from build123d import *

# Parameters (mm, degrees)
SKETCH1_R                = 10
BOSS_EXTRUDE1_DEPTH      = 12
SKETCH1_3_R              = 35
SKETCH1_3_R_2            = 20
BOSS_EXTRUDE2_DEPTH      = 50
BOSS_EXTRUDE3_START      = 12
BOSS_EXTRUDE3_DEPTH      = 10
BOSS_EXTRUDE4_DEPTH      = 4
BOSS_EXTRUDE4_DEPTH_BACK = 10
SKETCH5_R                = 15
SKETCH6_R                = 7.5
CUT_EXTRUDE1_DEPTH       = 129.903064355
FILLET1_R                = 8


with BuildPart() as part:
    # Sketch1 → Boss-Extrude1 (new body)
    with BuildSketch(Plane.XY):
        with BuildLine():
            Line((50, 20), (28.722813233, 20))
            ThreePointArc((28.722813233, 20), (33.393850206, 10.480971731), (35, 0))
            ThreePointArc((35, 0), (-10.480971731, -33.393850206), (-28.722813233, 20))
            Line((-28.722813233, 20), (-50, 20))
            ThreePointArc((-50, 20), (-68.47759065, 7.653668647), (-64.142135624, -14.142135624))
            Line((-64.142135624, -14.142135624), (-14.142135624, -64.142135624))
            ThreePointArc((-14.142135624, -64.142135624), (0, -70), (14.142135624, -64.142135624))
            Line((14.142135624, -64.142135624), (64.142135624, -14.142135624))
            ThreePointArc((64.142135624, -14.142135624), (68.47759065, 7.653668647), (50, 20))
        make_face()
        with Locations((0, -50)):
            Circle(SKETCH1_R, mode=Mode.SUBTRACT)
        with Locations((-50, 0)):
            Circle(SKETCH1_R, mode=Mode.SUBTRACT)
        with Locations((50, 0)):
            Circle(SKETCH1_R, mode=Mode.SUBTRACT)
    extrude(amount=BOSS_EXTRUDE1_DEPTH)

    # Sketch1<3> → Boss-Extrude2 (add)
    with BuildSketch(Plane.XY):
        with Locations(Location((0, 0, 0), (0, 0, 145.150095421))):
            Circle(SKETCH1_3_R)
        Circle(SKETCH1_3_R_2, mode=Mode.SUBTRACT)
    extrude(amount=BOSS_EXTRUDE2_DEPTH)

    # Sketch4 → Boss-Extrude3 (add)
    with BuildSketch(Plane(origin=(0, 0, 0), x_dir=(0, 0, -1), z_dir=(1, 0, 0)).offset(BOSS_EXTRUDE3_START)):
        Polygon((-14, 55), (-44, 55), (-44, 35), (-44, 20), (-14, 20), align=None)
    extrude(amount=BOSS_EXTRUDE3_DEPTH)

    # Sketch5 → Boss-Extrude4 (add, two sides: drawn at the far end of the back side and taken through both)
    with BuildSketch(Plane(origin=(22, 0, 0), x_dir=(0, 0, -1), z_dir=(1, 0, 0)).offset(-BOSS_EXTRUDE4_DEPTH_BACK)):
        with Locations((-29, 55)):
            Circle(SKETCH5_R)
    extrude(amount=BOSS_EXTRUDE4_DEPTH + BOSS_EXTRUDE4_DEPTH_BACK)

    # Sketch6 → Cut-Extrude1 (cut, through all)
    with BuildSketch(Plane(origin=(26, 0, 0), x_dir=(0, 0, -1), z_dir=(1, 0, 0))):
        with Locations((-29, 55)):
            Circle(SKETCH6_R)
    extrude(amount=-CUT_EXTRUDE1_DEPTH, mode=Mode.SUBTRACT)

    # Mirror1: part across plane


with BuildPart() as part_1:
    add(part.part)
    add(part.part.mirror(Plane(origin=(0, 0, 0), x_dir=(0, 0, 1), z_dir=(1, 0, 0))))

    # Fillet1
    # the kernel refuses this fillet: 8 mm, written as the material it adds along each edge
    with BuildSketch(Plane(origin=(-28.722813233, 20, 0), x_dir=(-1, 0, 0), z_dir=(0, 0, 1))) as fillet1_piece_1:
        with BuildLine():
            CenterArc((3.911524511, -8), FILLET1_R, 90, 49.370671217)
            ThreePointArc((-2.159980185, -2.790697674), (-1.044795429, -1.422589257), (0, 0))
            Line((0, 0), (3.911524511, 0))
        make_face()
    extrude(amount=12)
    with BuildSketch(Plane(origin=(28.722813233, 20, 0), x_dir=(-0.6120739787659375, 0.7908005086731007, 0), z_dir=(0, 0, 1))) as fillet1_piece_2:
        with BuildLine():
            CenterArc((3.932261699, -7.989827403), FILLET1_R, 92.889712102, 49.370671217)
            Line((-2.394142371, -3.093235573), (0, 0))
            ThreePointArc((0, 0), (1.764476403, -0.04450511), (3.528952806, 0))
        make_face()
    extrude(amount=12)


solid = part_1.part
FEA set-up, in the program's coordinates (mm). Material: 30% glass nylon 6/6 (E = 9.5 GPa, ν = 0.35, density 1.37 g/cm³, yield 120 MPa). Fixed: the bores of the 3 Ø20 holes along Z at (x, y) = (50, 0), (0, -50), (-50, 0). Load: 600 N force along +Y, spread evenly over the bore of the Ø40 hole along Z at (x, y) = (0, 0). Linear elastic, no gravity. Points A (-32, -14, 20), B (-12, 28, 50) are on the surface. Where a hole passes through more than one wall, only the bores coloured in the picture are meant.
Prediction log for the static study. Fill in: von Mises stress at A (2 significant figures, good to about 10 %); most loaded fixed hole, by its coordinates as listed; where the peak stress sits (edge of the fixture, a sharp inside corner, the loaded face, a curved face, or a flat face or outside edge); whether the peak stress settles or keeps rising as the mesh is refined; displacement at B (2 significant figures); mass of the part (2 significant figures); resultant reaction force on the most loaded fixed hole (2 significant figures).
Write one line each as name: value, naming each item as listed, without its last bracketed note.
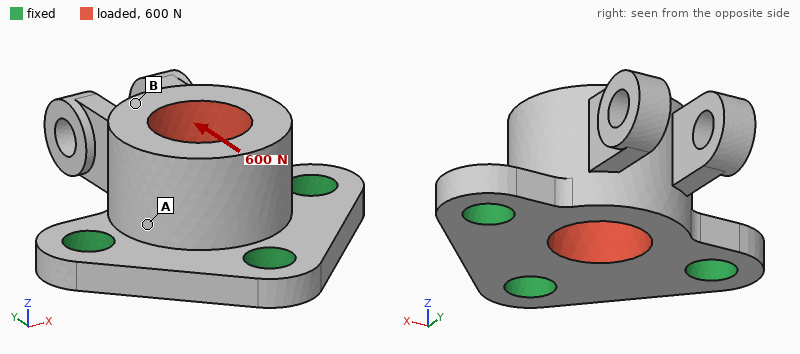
von Mises stress at A: 0.63 MPa
most loaded fixed hole, by its coordinates as listed: (0, -50)
where the peak stress sits: edge of the fixture
whether the peak stress settles or keeps rising as the mesh is refined: keeps rising
displacement at B: 15 µm
mass of the part: 280 g
resultant reaction force on the most loaded fixed hole: 360 N
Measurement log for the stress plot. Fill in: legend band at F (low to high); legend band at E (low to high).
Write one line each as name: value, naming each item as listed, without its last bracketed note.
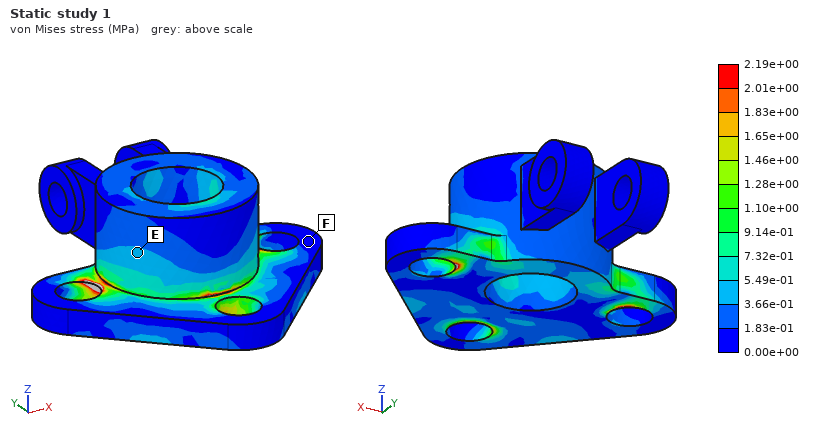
legend band at F: 0.00e+00 to 1.83e-01 MPa
legend band at E: 3.66e-01 to 5.49e-01 MPa
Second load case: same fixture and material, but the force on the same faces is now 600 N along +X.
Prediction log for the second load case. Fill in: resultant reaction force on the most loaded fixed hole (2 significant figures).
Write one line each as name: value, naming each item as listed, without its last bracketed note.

resultant reaction force on the most loaded fixed hole: 290 N
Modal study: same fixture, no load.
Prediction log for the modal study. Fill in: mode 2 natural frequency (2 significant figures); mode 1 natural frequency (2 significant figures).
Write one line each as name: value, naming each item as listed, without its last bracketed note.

mode 2 natural frequency: 2400 Hz
mode 1 natural frequency: 1800 Hz
